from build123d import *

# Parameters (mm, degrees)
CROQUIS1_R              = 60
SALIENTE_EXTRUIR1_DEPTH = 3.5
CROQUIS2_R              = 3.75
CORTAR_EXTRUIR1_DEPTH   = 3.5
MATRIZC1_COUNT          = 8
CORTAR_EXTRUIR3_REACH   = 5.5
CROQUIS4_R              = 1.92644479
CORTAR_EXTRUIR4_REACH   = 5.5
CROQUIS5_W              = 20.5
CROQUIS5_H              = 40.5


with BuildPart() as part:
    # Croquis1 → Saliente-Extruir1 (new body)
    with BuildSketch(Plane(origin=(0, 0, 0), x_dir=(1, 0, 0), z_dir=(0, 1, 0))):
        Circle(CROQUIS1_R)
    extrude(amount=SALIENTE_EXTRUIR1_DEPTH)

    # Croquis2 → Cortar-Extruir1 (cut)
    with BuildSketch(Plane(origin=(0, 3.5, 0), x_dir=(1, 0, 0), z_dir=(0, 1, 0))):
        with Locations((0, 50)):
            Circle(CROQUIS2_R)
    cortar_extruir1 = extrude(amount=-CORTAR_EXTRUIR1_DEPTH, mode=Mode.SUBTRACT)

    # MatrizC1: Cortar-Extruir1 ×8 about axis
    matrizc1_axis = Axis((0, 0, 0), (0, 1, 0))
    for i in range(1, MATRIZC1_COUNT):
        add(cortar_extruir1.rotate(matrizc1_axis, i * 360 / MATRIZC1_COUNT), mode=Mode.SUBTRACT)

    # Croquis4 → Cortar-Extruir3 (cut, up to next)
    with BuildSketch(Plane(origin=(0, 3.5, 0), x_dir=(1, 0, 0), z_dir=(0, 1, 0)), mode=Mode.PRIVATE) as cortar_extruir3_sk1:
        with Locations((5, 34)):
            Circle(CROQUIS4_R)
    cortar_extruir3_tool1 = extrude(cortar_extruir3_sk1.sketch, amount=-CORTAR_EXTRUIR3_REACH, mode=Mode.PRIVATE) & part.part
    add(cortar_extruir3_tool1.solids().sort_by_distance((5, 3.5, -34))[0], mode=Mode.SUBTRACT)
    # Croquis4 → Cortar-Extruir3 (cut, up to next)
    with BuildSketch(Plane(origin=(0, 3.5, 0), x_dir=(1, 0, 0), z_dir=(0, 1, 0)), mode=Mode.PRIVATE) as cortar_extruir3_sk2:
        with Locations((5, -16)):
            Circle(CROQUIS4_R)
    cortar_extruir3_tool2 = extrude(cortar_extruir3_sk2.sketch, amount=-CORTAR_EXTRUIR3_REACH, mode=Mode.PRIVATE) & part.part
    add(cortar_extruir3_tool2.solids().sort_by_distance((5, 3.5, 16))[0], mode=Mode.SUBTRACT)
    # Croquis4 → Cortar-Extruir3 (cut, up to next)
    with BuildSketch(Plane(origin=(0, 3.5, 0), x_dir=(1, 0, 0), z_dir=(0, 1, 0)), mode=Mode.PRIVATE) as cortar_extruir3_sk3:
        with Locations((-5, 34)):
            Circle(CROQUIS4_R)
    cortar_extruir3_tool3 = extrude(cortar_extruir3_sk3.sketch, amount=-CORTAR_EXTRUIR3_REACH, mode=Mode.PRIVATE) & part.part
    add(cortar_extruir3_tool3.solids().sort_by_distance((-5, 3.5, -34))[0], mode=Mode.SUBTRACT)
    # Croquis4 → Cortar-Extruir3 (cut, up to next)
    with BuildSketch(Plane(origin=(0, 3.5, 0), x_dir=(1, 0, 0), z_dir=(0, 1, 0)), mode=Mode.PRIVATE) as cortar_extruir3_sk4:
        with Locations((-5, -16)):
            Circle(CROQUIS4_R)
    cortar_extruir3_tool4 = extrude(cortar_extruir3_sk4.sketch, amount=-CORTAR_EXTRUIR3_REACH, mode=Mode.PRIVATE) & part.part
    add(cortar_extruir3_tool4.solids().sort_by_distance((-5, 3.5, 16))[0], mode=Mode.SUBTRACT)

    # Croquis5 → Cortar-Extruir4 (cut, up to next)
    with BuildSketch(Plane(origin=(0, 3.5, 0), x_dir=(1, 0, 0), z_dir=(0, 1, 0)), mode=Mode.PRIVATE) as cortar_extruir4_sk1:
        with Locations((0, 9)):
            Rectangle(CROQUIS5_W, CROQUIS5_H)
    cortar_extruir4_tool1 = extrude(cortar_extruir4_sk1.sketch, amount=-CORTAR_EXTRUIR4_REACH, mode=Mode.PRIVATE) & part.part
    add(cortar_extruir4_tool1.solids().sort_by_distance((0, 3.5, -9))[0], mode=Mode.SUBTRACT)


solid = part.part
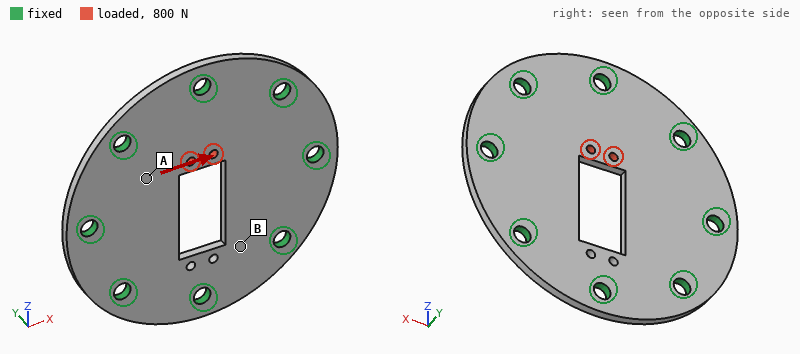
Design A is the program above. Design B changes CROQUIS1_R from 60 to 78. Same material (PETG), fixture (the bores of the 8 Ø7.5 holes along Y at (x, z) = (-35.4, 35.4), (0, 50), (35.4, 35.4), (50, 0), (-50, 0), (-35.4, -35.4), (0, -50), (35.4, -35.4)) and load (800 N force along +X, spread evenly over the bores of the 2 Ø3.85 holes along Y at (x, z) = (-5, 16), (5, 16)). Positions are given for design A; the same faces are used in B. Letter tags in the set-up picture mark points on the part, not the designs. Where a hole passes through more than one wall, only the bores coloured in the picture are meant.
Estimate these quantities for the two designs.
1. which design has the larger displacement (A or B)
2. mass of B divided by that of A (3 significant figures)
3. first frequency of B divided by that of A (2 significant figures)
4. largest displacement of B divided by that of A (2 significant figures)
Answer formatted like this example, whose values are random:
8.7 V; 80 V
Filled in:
A; 1.77; 0.47; 0.66
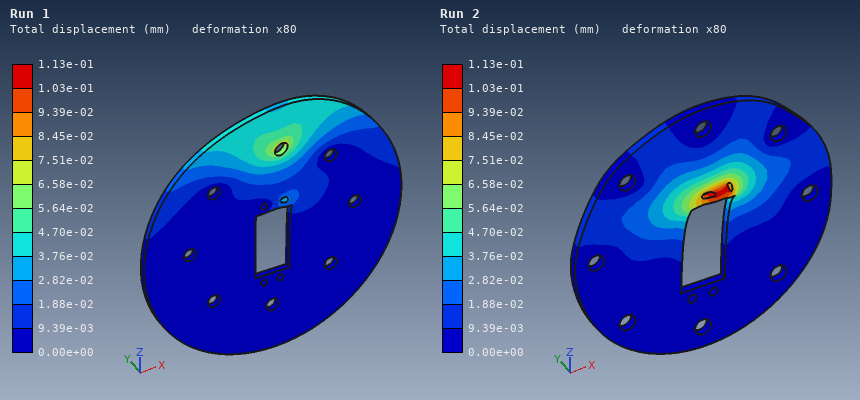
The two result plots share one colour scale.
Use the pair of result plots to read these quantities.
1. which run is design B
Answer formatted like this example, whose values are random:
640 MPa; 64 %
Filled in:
Run 1
